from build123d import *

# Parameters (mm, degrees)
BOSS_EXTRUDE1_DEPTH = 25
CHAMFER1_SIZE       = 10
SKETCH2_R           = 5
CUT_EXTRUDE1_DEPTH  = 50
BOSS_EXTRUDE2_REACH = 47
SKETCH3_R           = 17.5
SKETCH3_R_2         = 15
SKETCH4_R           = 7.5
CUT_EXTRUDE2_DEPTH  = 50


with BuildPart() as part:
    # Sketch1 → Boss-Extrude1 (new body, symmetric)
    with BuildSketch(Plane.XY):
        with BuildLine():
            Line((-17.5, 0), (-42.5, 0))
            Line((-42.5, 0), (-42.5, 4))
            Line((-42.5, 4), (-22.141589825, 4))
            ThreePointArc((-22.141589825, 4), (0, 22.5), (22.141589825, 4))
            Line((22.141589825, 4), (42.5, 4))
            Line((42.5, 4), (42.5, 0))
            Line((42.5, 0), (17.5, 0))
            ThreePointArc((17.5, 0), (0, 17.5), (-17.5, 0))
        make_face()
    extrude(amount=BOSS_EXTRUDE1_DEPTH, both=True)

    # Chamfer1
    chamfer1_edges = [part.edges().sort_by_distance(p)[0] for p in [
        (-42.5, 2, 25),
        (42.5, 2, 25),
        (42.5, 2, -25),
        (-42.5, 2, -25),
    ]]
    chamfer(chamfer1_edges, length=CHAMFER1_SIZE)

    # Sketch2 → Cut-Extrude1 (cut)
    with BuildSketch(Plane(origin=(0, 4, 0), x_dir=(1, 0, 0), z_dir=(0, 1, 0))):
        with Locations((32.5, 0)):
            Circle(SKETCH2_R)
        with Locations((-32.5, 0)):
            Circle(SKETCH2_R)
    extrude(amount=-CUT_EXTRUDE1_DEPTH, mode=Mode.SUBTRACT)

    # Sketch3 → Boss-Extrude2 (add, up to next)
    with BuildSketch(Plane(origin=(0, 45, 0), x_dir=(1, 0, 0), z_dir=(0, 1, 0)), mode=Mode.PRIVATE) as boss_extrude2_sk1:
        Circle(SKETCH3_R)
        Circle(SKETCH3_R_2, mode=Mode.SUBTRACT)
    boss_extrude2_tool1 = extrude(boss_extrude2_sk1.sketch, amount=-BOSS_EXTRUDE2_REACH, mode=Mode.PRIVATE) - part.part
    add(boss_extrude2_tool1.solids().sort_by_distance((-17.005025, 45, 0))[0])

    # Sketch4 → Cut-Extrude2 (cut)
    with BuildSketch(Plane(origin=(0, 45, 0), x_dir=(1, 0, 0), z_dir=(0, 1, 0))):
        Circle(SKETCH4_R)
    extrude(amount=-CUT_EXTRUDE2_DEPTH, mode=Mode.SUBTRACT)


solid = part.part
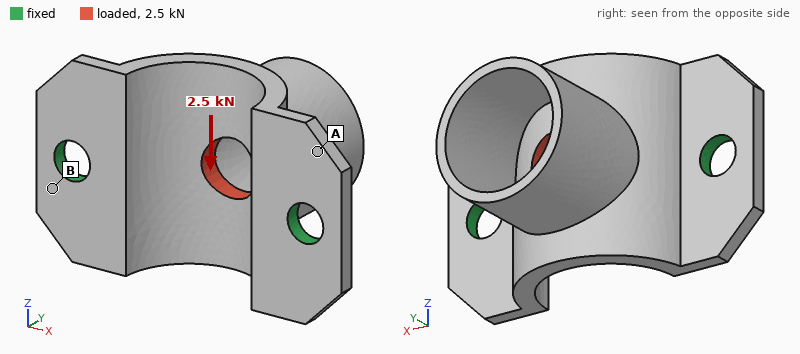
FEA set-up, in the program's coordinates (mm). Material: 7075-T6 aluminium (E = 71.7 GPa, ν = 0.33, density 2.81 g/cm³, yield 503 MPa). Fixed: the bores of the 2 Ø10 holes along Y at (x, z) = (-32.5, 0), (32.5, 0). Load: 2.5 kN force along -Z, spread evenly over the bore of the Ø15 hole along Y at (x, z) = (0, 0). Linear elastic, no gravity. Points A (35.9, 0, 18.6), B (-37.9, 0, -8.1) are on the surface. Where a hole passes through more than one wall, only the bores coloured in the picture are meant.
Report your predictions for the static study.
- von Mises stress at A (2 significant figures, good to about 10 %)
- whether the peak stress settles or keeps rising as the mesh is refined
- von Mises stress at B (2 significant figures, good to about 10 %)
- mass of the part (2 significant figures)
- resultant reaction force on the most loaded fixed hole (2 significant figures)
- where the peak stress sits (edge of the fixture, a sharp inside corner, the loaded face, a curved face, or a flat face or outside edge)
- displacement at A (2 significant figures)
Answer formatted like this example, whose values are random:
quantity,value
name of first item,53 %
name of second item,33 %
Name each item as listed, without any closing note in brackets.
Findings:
quantity,value
von Mises stress at A,35 MPa
whether the peak stress settles or keeps rising as the mesh is refined,keeps rising
von Mises stress at B,79 MPa
mass of the part,79 g
resultant reaction force on the most loaded fixed hole,1.3 kN
where the peak stress sits,edge of the fixture
displacement at A,0.049 mm
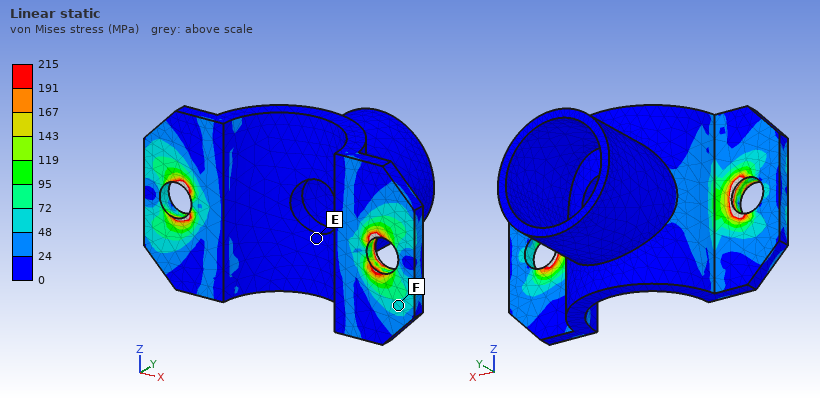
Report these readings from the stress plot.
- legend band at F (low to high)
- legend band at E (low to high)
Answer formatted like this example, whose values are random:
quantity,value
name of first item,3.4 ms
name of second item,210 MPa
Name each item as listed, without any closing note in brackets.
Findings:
quantity,value
legend band at F,48 to 72 MPa
legend band at E,0 to 24 MPa
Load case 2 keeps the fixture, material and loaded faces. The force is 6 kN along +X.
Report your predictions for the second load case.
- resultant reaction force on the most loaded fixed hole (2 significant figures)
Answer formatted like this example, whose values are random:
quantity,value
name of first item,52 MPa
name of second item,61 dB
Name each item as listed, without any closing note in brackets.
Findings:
quantity,value
resultant reaction force on the most loaded fixed hole,3.5 kN
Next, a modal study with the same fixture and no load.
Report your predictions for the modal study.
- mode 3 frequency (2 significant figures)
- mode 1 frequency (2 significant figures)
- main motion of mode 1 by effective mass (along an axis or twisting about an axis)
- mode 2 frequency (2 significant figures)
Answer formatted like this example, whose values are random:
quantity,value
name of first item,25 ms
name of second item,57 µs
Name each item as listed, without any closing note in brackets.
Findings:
quantity,value
mode 3 frequency,7400 Hz
mode 1 frequency,2300 Hz
main motion of mode 1 by effective mass,along Z
mode 2 frequency,7300 Hz
